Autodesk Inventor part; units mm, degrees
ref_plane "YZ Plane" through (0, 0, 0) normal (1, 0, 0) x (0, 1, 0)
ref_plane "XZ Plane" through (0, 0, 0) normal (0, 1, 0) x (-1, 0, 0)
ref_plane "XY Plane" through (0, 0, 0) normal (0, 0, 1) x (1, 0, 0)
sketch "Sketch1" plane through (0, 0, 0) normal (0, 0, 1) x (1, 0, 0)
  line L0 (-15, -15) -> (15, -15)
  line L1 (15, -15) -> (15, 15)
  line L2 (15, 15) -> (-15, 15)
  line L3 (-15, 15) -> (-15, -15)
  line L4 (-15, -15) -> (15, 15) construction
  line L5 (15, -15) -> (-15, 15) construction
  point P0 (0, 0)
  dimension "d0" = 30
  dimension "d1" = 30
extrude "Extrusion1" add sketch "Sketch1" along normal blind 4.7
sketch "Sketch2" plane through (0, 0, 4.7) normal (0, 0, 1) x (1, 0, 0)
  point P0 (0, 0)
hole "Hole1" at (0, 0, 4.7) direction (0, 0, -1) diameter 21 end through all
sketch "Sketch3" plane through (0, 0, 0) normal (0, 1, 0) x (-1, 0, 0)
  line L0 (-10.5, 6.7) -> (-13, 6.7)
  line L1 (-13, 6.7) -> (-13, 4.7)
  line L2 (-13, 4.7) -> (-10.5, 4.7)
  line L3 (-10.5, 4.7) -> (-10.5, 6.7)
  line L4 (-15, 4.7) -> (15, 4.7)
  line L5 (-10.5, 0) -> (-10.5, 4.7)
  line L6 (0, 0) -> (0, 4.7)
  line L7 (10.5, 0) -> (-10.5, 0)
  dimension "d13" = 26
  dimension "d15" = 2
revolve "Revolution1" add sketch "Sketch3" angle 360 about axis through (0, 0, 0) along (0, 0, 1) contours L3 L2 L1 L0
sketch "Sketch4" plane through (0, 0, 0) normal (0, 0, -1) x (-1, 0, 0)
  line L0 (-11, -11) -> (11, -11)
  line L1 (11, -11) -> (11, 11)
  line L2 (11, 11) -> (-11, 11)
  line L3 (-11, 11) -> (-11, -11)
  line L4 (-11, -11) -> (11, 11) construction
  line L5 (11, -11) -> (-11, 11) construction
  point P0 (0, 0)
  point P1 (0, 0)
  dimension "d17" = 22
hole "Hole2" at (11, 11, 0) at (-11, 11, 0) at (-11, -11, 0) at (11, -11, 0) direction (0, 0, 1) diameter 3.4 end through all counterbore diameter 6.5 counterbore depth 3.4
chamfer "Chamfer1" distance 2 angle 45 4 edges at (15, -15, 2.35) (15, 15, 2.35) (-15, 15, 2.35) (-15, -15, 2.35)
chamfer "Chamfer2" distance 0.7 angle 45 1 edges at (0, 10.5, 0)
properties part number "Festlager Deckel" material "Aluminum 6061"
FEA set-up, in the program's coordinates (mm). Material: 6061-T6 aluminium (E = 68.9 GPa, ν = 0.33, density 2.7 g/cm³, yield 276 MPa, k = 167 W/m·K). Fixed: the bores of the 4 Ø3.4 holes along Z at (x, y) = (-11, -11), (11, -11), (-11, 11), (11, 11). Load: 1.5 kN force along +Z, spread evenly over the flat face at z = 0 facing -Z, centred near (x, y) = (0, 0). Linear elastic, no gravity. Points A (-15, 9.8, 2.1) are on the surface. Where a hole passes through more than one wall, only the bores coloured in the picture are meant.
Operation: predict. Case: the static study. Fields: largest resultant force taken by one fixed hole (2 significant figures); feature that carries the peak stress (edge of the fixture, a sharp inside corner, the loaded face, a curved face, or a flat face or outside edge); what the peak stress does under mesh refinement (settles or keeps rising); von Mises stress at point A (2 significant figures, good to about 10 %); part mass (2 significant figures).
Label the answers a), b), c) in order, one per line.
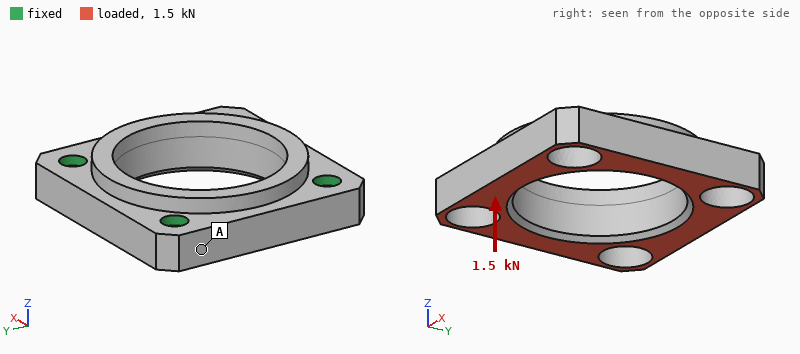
a) 380 N
b) edge of the fixture
c) keeps rising
d) 14 MPa
e) 6.5 g
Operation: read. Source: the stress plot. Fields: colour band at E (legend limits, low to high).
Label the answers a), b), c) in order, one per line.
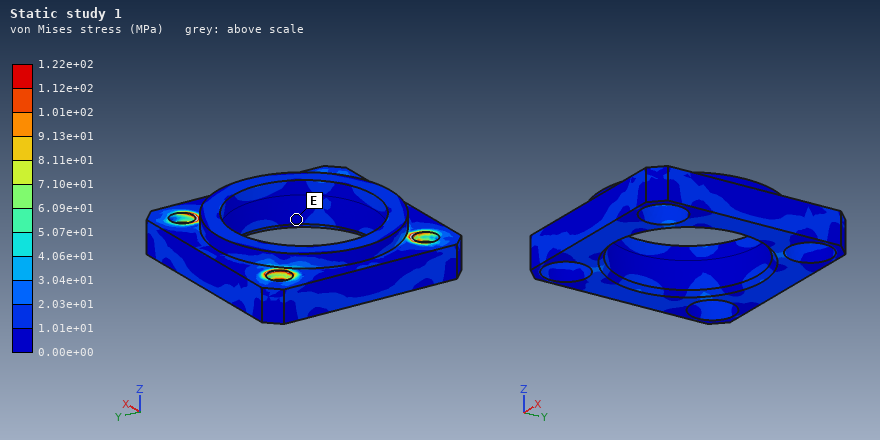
a) 0.00e+00 to 1.01e+01 MPa
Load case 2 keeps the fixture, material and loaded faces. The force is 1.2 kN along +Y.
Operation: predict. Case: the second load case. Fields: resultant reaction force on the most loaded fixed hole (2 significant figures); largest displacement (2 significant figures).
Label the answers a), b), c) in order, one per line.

a) 320 N
b) 8.8 µm
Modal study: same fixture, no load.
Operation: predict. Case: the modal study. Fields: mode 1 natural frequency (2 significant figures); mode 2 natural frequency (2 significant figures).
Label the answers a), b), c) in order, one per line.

a) 25 kHz
b) 31 kHz
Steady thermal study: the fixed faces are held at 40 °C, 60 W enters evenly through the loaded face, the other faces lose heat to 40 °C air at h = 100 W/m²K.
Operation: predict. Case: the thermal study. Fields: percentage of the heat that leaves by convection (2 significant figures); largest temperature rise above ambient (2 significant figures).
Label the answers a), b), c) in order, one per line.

a) 3.9 %
b) 17 K
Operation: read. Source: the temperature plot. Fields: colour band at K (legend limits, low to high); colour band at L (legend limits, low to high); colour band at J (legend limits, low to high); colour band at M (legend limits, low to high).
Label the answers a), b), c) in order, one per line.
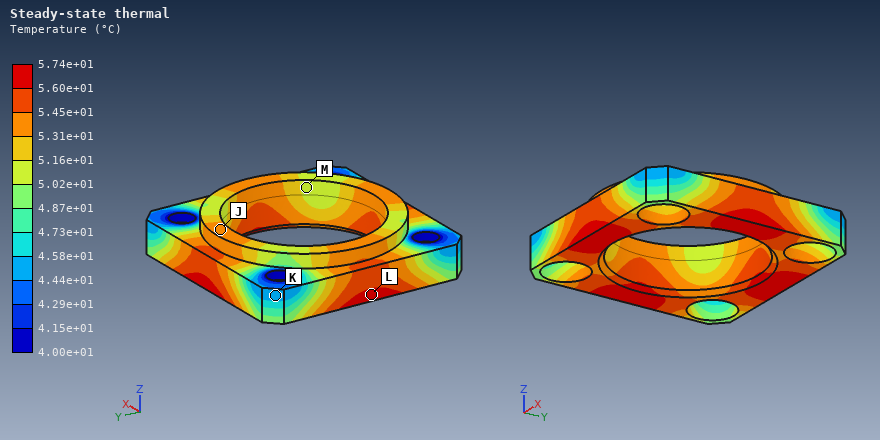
a) 4.44e+01 to 4.58e+01 °C
b) 5.60e+01 to 5.74e+01 °C
c) 5.31e+01 to 5.45e+01 °C
d) 5.02e+01 to 5.16e+01 °C
